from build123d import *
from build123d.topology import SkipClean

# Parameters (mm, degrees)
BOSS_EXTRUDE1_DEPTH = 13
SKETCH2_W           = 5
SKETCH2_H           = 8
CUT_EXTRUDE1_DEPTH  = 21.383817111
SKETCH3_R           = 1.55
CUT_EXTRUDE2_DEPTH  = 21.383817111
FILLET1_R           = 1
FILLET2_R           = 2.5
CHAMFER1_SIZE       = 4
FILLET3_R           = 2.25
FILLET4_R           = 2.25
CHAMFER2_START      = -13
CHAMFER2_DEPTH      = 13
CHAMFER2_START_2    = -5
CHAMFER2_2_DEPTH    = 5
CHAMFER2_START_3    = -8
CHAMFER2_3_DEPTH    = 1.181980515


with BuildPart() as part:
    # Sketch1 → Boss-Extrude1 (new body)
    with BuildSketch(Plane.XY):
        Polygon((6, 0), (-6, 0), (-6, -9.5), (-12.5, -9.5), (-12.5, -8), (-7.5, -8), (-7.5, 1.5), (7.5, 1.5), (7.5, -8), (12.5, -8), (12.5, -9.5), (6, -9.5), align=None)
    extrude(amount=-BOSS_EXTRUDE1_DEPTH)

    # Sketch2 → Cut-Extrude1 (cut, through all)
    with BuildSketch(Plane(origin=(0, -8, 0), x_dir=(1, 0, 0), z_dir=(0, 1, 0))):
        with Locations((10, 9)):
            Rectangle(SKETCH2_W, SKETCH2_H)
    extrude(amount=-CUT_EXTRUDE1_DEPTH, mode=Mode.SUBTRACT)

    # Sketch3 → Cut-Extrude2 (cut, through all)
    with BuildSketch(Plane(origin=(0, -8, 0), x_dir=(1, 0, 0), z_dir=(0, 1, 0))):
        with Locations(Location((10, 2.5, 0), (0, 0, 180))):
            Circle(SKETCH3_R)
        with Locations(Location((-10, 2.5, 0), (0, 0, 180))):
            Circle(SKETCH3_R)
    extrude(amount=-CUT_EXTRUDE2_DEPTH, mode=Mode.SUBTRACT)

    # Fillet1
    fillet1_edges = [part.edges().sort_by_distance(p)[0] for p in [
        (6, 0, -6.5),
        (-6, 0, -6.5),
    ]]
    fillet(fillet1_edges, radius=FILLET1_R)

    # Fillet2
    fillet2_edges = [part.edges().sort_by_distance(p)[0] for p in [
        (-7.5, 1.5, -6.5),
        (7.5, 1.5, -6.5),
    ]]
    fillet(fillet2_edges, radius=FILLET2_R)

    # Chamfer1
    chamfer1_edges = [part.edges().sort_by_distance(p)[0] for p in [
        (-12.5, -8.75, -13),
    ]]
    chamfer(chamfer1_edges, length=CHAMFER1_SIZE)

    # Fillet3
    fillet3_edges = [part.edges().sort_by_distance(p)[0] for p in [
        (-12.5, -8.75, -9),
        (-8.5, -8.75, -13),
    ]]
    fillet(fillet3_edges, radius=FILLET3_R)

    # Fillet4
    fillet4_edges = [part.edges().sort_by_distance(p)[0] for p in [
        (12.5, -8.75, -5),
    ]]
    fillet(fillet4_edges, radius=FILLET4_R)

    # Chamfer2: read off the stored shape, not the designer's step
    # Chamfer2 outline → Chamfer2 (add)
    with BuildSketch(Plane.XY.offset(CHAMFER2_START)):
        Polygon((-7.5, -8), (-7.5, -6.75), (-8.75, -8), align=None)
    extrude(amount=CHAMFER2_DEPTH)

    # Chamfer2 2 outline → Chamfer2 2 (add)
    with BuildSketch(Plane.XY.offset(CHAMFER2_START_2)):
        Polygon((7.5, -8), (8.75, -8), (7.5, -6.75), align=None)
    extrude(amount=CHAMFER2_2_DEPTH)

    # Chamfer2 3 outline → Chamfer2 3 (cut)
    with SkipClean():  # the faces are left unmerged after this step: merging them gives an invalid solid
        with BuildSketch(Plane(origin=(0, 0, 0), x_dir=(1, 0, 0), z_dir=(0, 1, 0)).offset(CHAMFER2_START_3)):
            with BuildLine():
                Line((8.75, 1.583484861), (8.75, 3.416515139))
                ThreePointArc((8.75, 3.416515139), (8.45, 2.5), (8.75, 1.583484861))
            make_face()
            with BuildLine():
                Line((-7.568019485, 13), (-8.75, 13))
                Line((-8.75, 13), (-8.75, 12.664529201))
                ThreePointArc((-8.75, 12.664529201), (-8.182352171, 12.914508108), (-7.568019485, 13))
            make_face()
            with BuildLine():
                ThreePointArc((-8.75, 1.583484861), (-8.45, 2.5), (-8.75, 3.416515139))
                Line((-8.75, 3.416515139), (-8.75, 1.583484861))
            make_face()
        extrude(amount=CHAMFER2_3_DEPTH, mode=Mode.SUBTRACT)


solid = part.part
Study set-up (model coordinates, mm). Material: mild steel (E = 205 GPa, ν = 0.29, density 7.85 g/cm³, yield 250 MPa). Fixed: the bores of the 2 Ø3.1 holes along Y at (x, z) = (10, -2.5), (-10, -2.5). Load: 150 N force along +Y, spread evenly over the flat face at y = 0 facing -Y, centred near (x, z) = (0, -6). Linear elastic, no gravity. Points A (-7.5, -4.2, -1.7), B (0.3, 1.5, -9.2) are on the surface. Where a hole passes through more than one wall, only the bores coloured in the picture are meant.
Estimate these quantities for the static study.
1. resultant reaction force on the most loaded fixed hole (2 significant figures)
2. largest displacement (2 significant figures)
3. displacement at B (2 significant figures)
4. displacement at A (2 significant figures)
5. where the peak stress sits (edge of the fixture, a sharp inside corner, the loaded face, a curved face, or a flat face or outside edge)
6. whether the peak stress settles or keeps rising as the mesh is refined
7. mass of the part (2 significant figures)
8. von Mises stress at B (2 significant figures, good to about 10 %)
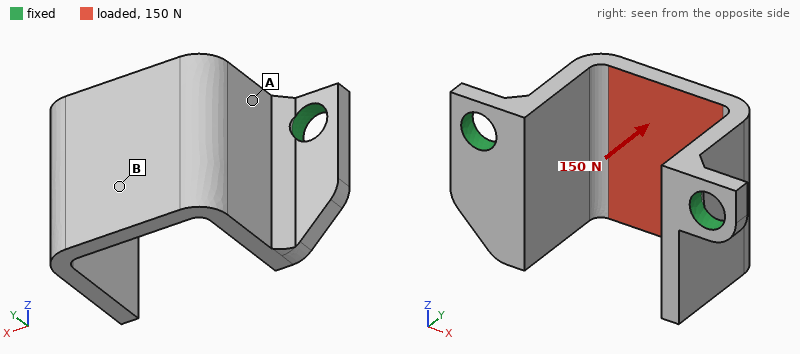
82 N
10 µm
8.3 µm
2.2 µm
edge of the fixture
keeps rising
5.9 g
29 MPa
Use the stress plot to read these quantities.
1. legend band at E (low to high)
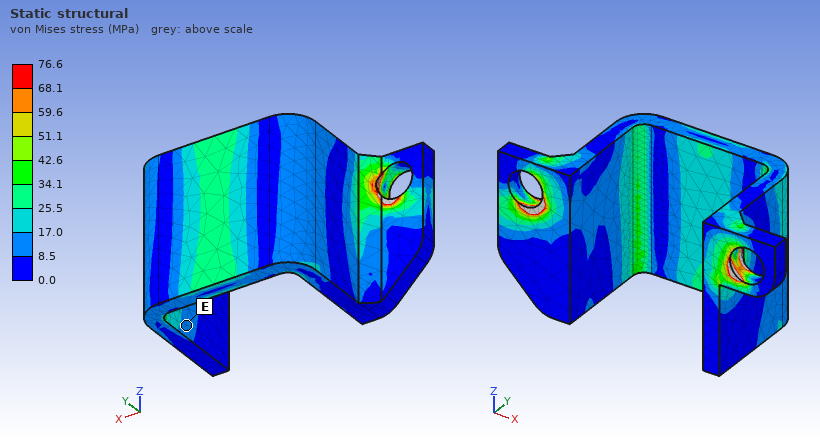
8.5 to 17.0 MPa
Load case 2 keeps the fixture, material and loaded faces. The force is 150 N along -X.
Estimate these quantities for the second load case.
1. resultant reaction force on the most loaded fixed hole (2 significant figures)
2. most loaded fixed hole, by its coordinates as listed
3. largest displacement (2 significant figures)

94 N
(-10, -2.5)
14 µm
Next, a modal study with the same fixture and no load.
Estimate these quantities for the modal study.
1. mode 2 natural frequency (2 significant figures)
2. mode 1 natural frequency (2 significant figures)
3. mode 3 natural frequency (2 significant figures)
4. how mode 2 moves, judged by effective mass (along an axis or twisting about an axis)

9700 Hz
8200 Hz
13 kHz
along X
